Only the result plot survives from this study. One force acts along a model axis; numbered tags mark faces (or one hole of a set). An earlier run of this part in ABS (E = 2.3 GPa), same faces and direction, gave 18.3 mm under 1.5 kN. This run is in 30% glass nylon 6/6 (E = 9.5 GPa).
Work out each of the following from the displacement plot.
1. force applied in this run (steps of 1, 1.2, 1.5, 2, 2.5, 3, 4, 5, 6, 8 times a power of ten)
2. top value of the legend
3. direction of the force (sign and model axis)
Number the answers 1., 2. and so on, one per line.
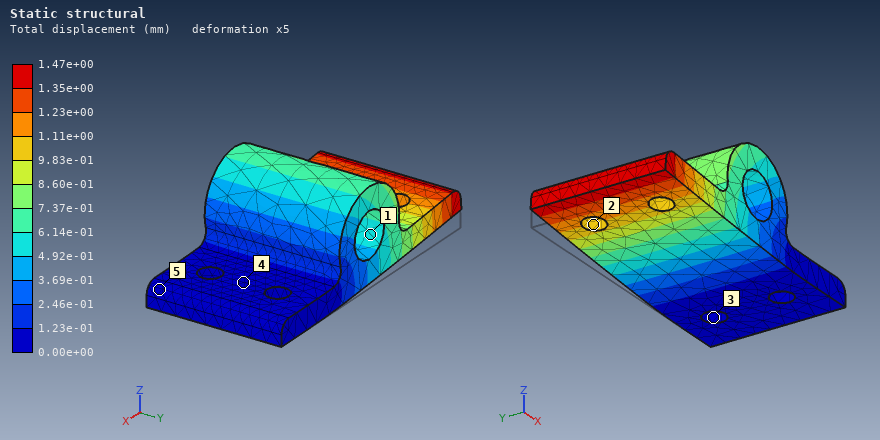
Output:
1. 500 N
2. 1.47e+00 mm
3. +Z
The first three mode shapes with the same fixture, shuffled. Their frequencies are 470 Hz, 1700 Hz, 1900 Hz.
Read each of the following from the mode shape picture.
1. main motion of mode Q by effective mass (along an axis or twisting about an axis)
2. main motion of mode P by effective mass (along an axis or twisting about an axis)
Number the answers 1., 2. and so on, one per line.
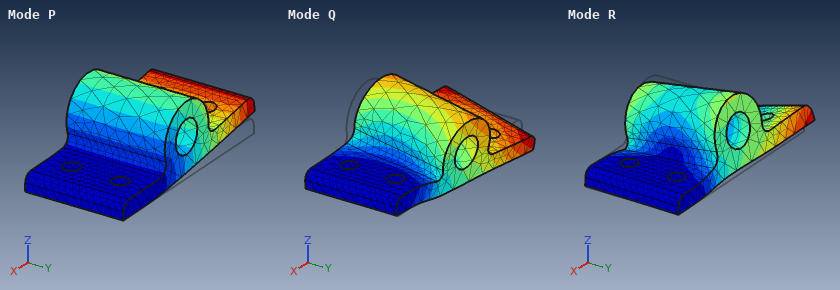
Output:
1. along Y
2. along Z
